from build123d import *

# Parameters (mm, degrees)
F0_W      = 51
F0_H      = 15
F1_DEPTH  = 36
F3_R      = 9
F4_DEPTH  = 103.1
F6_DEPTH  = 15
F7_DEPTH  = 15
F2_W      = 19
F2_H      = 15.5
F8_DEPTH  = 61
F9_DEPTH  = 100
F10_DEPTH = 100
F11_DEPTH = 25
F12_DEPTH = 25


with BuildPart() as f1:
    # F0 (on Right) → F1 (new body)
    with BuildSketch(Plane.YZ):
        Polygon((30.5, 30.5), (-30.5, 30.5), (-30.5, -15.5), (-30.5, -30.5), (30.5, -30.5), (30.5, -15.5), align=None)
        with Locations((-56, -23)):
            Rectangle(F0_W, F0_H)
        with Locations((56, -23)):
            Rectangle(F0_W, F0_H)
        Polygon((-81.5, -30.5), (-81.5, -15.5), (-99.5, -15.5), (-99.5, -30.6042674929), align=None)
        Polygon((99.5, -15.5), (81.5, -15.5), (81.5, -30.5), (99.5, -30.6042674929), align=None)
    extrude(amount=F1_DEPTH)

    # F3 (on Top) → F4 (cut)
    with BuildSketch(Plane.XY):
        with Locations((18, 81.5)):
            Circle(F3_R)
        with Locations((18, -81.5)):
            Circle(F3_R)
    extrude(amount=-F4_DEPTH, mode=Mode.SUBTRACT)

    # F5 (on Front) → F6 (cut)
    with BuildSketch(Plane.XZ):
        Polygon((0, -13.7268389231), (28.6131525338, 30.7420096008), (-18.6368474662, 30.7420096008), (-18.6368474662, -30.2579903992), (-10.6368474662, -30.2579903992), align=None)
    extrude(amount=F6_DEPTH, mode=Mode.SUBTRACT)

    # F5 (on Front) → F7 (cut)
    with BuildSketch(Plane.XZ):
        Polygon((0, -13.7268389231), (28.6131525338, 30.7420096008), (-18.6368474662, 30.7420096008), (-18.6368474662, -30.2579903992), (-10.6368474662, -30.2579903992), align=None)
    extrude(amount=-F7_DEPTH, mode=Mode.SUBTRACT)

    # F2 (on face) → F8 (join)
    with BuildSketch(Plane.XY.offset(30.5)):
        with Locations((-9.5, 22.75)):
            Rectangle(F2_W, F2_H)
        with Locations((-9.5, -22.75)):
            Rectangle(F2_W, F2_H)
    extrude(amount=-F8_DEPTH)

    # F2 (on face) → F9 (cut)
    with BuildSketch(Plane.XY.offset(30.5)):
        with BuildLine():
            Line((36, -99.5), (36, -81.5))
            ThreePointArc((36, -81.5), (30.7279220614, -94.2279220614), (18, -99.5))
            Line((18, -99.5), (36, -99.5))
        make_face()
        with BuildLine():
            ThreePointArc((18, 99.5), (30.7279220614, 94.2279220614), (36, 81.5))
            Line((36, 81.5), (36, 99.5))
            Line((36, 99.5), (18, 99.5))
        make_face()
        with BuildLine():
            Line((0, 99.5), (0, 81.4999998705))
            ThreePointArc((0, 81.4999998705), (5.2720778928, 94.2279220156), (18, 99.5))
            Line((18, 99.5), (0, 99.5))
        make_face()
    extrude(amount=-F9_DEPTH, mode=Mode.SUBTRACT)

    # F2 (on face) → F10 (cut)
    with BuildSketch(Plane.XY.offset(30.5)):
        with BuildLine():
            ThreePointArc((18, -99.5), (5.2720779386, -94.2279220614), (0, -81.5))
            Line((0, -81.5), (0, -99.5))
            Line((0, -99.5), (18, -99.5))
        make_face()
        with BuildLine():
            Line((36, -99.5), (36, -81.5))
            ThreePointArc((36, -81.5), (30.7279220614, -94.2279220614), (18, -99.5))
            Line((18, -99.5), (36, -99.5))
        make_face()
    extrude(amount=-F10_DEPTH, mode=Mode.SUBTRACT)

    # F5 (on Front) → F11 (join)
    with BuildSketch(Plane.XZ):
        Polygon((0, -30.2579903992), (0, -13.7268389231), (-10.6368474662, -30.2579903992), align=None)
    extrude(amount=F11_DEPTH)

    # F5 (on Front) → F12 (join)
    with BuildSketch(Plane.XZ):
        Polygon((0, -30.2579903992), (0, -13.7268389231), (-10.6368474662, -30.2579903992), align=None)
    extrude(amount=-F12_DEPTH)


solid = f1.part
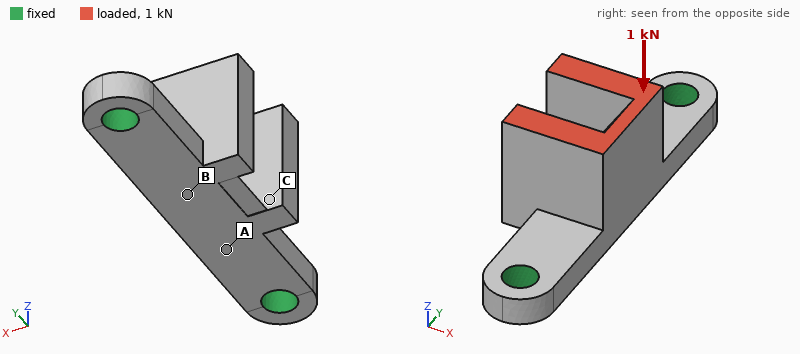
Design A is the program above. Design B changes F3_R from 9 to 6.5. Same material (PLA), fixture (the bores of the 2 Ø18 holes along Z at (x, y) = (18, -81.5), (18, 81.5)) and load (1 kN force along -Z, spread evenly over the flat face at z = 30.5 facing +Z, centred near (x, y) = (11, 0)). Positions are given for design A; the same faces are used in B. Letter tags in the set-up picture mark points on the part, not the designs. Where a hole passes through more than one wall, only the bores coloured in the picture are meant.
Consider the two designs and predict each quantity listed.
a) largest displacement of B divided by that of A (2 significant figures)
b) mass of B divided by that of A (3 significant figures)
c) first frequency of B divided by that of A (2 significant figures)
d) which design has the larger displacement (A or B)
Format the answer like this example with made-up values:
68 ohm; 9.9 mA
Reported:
1.1; 1.02; 0.95; B
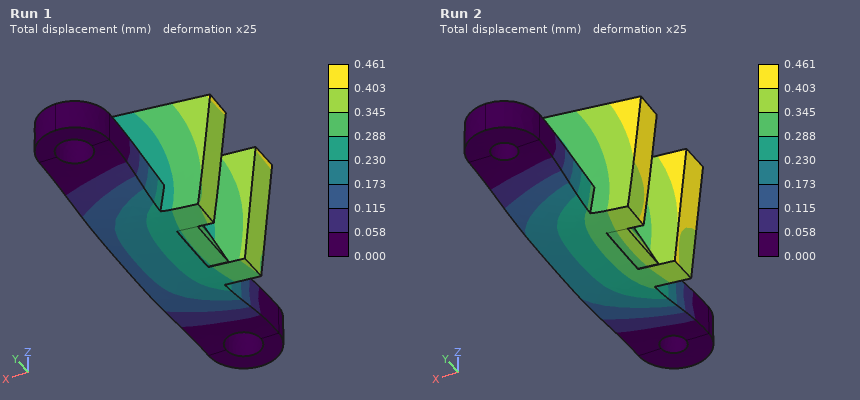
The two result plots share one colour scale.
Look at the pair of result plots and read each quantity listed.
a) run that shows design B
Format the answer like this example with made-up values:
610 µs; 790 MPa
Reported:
Run 2
